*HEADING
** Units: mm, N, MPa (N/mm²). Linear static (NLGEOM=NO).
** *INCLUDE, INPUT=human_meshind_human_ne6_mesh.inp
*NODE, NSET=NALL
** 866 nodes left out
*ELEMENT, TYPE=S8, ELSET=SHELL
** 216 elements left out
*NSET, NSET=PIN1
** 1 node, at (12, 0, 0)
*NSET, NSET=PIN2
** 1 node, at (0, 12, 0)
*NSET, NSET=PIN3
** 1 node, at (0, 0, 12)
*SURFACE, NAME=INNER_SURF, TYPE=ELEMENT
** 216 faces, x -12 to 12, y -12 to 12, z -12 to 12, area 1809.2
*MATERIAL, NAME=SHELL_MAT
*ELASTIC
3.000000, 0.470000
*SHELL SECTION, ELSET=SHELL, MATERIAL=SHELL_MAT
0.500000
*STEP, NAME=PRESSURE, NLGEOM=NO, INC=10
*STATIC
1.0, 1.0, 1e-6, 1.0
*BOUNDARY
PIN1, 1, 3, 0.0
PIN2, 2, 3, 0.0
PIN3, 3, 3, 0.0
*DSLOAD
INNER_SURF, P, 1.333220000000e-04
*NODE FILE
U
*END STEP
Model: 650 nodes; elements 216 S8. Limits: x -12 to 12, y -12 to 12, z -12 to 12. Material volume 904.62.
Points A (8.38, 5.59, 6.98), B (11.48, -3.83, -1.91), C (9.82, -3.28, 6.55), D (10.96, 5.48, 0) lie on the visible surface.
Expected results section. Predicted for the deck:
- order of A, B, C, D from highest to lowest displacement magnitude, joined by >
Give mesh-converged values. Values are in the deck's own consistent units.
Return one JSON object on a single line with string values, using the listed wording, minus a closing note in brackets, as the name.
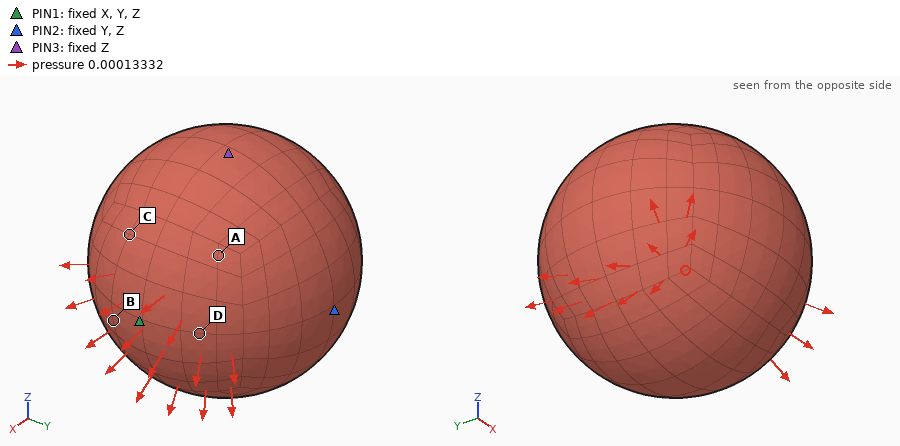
{"order of A, B, C, D from highest to lowest displacement magnitude, joined by >": "A > C > D > B"}
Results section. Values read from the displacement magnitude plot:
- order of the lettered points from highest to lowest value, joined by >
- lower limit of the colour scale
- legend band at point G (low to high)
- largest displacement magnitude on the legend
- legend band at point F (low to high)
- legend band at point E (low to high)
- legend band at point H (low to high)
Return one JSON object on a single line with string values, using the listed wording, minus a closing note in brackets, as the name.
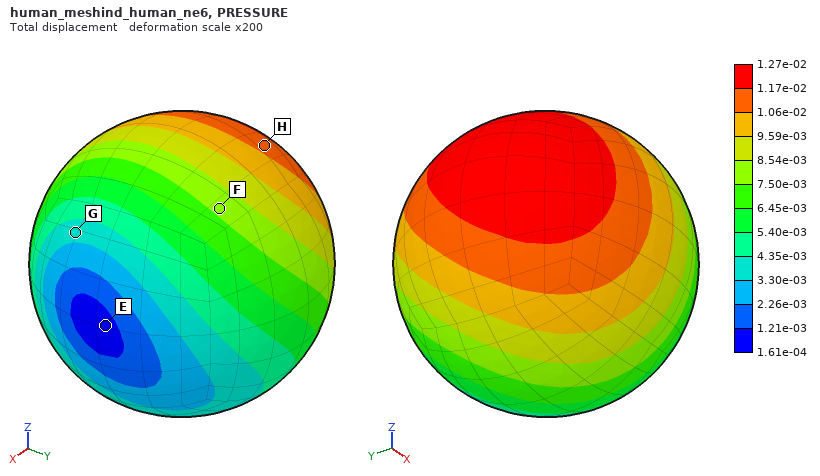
{"order of the lettered points from highest to lowest value, joined by >": "H > F > G > E", "lower limit of the colour scale": "1.61e-04", "legend band at point G": "3.30e-03 to 4.35e-03", "largest displacement magnitude on the legend": "1.27e-02", "legend band at point F": "7.50e-03 to 8.54e-03", "legend band at point E": "1.61e-04 to 1.21e-03", "legend band at point H": "1.06e-02 to 1.17e-02"}
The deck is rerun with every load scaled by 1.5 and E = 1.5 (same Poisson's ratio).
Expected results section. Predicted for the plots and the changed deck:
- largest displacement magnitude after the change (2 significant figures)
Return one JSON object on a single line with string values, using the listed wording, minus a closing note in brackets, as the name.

{"largest displacement magnitude after the change": "0.038"}
